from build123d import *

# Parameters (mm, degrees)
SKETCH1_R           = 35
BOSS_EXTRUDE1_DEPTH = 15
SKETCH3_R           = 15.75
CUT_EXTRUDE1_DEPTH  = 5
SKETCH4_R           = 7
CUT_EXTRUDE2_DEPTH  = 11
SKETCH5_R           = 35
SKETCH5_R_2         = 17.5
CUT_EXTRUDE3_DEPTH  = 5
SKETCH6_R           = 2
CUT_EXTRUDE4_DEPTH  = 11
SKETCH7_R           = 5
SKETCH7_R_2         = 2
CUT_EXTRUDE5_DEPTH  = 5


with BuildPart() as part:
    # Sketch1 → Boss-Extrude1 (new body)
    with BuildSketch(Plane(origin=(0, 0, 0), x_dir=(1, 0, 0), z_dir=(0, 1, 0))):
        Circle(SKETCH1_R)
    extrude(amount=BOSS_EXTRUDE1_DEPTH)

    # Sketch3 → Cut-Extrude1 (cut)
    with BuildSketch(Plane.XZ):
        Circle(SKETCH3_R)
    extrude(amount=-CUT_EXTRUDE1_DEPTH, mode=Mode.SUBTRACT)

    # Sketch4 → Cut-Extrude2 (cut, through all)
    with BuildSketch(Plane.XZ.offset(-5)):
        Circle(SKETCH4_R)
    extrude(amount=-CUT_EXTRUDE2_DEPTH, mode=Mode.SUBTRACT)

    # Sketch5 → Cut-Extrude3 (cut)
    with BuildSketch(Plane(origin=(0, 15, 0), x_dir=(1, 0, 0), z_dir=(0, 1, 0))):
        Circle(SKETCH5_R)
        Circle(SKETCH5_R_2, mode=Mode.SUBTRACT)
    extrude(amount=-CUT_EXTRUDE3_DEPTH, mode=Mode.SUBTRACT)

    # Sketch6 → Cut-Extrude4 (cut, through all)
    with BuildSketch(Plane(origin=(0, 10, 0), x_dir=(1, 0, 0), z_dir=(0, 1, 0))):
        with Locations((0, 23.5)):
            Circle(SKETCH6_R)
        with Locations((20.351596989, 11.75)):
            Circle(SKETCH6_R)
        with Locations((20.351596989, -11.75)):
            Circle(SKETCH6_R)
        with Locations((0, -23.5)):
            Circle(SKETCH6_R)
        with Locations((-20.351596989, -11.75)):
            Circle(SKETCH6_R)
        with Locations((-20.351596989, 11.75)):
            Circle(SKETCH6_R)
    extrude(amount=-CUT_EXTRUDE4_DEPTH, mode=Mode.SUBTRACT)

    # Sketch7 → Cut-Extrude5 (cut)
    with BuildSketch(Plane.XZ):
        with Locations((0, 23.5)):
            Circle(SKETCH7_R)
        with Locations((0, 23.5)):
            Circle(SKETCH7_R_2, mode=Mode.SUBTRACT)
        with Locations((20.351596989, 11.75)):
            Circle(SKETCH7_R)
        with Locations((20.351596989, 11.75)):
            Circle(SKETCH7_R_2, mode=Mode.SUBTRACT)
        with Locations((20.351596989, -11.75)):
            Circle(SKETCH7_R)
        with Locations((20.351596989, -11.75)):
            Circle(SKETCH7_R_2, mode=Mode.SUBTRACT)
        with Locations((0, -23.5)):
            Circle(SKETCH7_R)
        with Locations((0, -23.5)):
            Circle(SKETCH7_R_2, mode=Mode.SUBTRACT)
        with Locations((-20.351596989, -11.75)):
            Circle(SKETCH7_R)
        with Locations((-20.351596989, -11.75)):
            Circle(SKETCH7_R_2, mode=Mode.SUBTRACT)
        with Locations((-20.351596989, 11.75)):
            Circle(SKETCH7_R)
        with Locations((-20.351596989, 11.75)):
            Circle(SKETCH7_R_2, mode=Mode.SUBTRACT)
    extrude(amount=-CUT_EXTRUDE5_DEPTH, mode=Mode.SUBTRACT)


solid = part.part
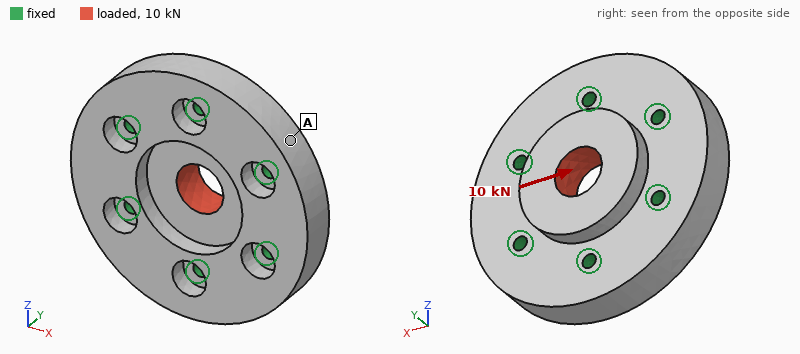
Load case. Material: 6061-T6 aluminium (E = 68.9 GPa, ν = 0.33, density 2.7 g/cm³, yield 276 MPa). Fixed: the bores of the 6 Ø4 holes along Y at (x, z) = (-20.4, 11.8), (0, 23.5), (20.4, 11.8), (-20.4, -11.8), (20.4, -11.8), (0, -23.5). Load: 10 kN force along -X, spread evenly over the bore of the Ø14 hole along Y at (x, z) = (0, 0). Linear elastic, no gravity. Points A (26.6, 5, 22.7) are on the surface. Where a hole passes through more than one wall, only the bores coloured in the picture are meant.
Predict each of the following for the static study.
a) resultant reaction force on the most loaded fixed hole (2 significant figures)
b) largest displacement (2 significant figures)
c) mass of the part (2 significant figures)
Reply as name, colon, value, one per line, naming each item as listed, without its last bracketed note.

resultant reaction force on the most loaded fixed hole: 2.1 kN
largest displacement: 9.5 µm
mass of the part: 95 g
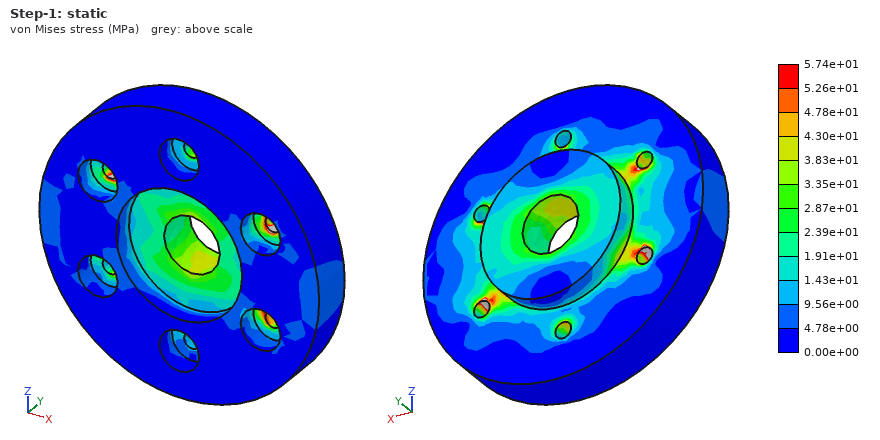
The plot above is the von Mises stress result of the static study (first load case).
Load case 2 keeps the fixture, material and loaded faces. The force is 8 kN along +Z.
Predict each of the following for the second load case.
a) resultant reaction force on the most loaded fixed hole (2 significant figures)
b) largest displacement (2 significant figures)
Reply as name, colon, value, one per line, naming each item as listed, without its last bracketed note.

resultant reaction force on the most loaded fixed hole: 1.9 kN
largest displacement: 7.6 µm
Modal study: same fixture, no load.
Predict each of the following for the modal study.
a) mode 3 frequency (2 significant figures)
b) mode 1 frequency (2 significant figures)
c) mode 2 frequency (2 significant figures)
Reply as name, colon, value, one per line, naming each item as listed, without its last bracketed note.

mode 3 frequency: 20 kHz
mode 1 frequency: 19 kHz
mode 2 frequency: 20 kHz
